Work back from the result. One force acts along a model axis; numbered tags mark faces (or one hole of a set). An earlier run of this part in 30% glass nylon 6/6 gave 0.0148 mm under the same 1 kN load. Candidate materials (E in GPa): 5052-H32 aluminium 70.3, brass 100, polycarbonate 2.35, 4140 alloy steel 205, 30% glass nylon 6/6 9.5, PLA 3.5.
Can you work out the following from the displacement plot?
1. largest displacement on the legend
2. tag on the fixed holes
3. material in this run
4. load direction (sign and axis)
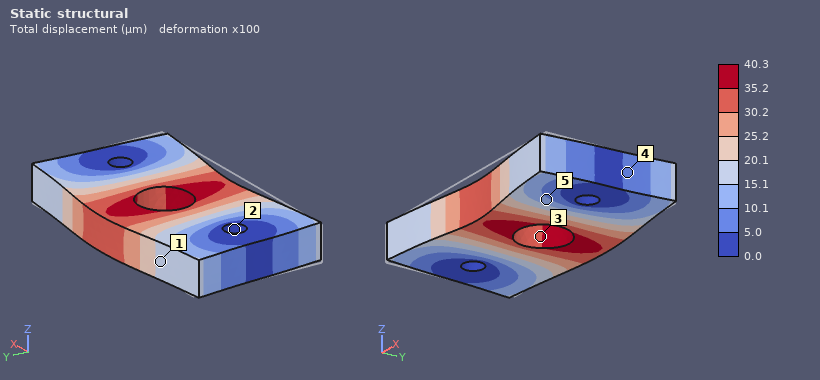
40.3 µm
2
PLA
+Y
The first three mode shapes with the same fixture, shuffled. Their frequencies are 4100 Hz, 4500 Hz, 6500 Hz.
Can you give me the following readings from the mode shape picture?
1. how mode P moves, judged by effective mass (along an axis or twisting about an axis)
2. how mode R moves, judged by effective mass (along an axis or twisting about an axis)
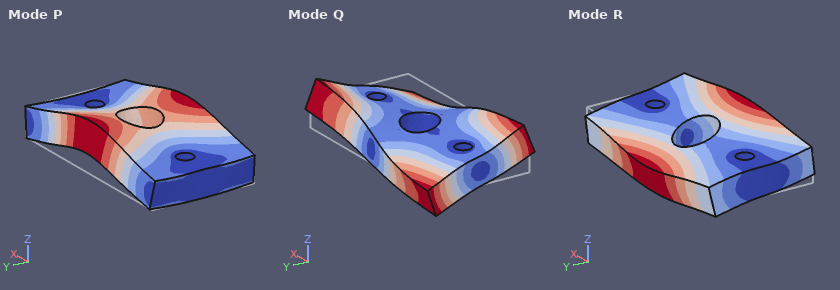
along Z
twisting about X
